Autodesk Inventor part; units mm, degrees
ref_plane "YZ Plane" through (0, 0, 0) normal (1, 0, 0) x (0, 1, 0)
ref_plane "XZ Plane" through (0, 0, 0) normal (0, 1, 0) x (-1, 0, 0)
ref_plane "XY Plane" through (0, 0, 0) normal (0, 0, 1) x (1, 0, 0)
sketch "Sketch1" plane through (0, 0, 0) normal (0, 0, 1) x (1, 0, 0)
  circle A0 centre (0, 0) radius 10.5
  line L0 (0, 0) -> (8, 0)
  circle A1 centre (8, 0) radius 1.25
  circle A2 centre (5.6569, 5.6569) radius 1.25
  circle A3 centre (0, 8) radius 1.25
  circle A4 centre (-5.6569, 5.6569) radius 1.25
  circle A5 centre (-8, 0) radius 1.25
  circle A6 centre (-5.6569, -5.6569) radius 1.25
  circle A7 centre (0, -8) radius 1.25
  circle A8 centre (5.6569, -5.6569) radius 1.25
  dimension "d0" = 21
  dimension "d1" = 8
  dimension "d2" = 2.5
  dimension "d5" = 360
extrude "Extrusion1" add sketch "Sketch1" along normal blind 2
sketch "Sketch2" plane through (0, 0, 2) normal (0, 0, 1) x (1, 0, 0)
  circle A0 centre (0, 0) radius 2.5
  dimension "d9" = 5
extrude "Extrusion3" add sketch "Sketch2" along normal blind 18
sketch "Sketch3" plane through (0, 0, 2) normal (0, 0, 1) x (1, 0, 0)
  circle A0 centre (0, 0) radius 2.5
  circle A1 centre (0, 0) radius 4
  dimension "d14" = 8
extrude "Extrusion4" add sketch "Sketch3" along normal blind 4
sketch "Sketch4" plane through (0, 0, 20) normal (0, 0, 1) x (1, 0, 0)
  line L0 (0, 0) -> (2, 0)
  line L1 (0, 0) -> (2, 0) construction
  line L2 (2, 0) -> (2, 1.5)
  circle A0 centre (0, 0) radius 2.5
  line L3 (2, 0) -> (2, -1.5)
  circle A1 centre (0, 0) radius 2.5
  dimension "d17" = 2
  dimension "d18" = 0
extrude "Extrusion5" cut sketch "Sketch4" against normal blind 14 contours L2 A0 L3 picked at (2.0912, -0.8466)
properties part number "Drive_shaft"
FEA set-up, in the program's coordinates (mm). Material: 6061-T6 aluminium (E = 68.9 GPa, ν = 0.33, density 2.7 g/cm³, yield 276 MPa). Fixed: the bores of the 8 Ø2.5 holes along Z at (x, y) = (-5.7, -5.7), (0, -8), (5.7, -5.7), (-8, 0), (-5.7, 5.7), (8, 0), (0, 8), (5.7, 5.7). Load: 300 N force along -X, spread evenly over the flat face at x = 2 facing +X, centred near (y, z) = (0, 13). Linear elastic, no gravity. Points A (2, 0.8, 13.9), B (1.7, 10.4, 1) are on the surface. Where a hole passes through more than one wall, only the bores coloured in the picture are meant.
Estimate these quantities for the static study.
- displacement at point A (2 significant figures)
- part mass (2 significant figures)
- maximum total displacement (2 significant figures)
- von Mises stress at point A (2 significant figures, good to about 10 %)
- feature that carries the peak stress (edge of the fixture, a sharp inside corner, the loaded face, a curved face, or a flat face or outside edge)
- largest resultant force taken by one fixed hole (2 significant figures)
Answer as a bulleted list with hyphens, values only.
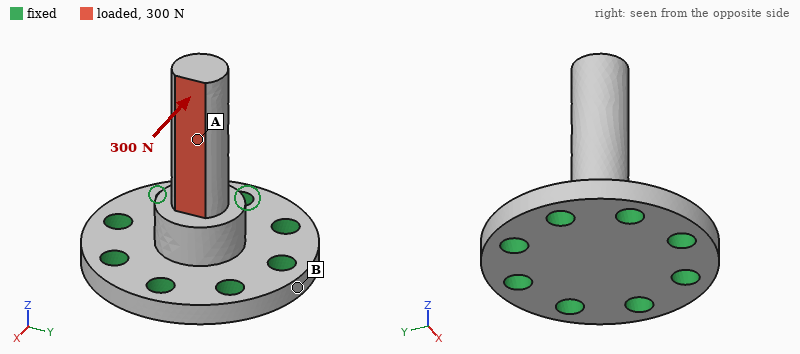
- 0.065 mm
- 2.9 g
- 0.12 mm
- 36 MPa
- the loaded face
- 170 N
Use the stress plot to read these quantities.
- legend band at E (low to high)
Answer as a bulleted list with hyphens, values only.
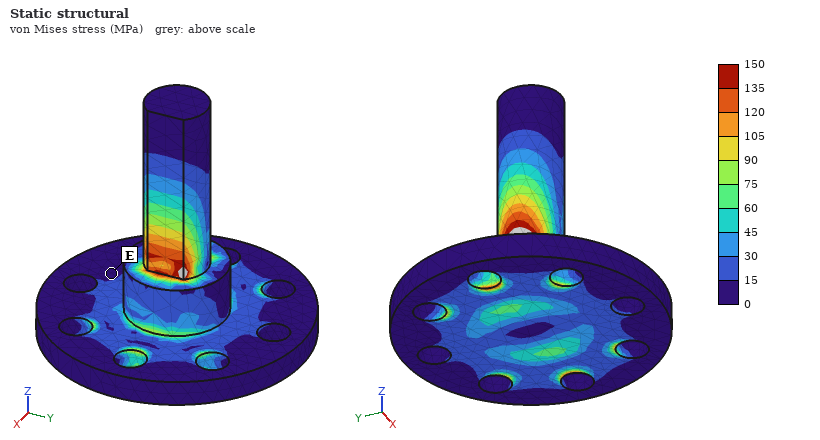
- 0 to 15 MPa
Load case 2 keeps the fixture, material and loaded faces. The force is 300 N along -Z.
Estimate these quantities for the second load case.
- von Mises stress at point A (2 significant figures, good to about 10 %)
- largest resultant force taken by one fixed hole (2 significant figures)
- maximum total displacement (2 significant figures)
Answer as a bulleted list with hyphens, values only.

- 32 MPa
- 66 N
- 36 µm
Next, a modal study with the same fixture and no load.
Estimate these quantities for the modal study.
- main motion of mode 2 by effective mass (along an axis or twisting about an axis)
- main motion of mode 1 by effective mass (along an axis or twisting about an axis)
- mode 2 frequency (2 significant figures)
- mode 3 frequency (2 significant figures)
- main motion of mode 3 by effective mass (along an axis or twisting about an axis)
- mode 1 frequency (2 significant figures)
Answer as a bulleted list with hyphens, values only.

- along Y
- along X
- 12 kHz
- 45 kHz
- along Z
- 12 kHz
